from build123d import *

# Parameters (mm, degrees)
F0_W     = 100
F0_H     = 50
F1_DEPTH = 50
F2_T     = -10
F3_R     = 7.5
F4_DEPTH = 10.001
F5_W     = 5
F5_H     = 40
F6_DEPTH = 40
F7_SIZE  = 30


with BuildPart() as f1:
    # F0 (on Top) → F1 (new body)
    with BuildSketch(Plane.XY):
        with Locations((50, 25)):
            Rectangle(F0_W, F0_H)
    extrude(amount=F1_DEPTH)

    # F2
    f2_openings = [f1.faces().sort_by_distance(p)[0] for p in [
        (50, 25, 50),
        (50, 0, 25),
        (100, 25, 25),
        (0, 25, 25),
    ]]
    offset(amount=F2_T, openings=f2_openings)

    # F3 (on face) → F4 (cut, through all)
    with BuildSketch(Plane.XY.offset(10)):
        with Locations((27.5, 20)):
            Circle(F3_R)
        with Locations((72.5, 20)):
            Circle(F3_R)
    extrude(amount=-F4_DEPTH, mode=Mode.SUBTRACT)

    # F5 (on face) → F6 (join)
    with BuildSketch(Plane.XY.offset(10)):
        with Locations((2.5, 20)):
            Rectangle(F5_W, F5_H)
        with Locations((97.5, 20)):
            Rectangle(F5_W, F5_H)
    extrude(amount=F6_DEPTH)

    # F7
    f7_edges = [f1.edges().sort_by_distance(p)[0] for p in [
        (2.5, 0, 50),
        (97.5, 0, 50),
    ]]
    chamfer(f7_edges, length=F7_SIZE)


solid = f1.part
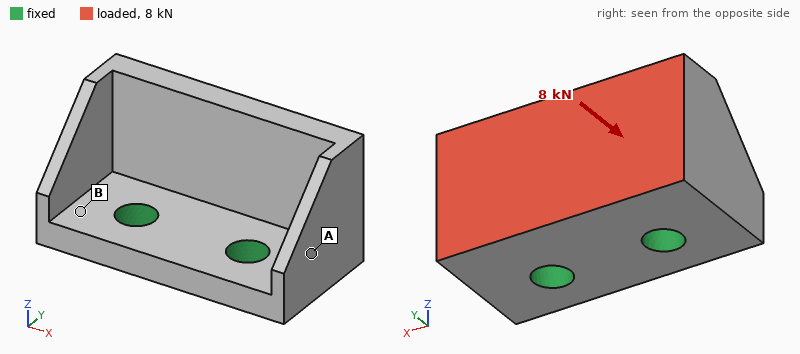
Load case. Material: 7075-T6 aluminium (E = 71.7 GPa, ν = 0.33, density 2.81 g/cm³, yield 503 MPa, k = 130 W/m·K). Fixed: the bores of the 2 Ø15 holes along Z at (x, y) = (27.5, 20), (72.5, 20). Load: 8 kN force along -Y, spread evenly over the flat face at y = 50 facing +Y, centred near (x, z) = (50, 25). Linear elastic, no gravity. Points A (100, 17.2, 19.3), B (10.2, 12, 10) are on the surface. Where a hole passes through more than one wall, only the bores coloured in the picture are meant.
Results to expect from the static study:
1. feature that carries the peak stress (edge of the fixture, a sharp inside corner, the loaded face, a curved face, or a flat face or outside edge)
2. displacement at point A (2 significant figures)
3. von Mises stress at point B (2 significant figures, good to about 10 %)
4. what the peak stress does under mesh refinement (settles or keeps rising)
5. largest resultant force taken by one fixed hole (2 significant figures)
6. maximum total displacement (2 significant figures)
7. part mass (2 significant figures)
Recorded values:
edge of the fixture
0.046 mm
46 MPa
keeps rising
4.0 kN
0.20 mm
280 g
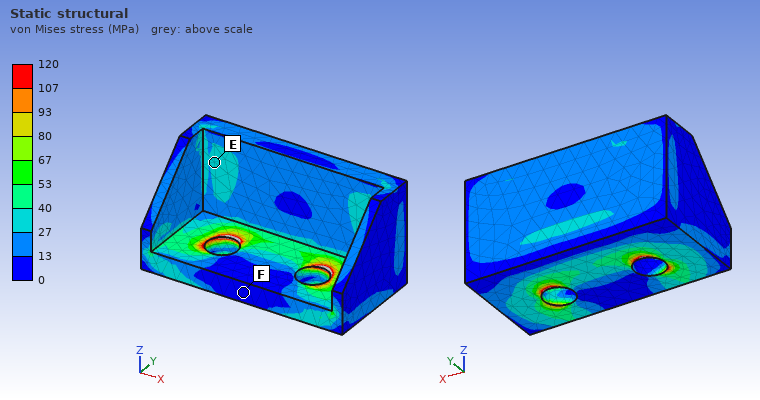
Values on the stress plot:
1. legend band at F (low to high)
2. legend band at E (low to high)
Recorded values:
0 to 13 MPa
27 to 40 MPa
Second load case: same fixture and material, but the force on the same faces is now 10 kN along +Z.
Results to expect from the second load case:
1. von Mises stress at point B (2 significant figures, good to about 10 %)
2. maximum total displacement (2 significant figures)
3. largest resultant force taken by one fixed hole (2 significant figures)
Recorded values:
49 MPa
0.21 mm
5.0 kN
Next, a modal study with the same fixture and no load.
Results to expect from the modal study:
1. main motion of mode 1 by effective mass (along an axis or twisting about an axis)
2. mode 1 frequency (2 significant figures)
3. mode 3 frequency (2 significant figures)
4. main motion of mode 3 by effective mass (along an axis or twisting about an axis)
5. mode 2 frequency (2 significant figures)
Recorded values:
along Y
3000 Hz
6400 Hz
along X
3600 Hz
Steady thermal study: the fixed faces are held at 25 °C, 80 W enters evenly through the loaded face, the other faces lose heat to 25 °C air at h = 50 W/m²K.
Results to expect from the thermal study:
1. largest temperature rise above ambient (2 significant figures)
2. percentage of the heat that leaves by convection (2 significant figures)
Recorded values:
20 K
12 %
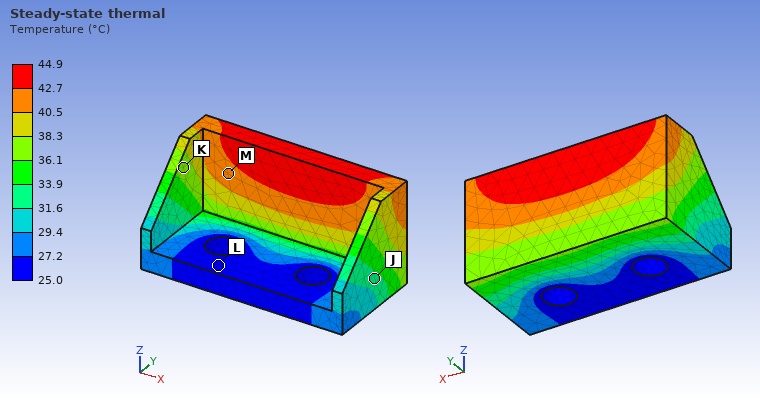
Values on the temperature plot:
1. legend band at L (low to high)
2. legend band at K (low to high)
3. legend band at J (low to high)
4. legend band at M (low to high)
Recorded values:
25.0 to 27.2 °C
36.1 to 38.3 °C
31.6 to 33.9 °C
40.5 to 42.7 °C
